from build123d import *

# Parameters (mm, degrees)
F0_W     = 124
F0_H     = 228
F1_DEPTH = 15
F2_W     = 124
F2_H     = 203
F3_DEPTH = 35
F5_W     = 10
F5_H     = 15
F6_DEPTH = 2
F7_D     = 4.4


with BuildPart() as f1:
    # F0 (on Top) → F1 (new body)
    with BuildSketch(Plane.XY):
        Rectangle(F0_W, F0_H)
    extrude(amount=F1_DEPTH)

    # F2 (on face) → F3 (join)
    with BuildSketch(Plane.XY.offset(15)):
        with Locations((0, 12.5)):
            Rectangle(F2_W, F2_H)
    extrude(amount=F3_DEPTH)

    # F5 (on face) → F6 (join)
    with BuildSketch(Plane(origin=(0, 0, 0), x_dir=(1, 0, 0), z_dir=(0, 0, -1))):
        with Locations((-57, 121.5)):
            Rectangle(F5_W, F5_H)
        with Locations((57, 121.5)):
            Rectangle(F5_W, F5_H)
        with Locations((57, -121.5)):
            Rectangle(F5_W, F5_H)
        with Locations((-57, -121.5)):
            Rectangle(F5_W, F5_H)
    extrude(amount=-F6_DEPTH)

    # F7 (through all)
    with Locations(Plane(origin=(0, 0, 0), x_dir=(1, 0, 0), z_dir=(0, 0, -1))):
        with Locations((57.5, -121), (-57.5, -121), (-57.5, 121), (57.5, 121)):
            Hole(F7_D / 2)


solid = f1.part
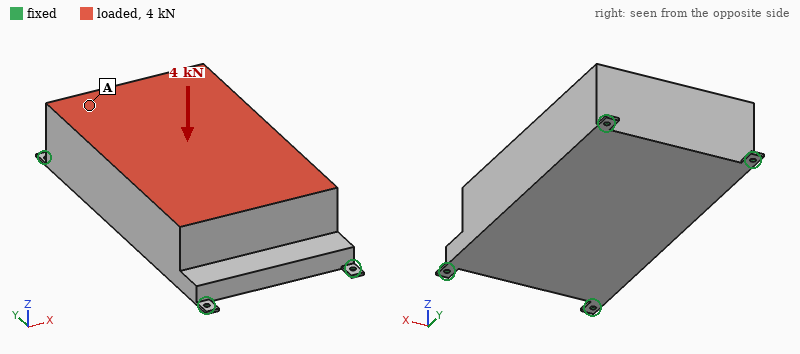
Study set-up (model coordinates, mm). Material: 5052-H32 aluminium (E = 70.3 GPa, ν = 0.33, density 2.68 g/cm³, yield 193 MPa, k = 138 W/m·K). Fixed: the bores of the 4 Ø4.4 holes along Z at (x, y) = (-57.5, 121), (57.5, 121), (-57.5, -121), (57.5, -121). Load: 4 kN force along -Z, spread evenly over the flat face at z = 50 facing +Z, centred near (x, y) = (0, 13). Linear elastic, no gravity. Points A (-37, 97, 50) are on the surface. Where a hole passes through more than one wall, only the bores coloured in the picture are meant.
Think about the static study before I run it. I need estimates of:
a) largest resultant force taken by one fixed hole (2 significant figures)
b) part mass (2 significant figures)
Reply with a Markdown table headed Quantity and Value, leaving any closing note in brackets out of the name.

| Quantity | Value |
|---|---|
| largest resultant force taken by one fixed hole | 1.4 kN |
| part mass | 3.5 kg |
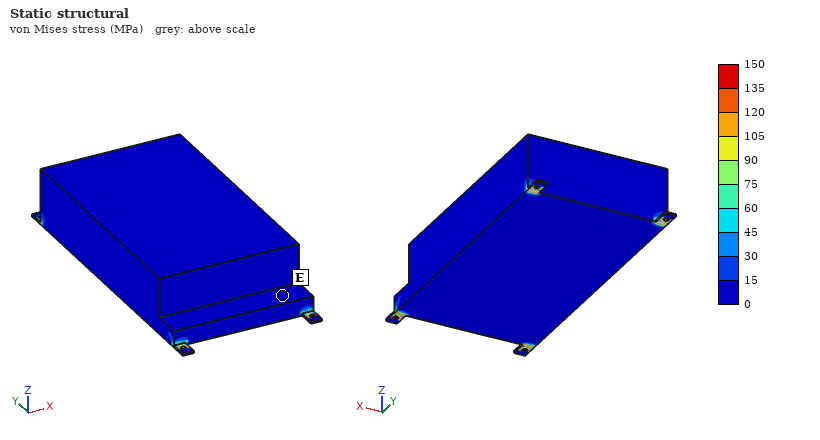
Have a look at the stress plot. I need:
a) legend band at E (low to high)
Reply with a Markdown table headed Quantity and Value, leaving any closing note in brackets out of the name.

| Quantity | Value |
|---|---|
| legend band at E | 0 to 15 MPa |
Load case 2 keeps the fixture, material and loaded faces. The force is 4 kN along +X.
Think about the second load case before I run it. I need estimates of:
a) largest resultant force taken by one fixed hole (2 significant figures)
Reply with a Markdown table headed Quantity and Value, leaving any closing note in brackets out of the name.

| Quantity | Value |
|---|---|
| largest resultant force taken by one fixed hole | 1.6 kN |
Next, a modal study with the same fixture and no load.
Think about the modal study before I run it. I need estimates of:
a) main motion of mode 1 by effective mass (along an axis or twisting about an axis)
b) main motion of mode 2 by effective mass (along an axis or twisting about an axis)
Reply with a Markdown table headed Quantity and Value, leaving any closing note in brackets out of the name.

| Quantity | Value |
|---|---|
| main motion of mode 1 by effective mass | along Z |
| main motion of mode 2 by effective mass | along X |
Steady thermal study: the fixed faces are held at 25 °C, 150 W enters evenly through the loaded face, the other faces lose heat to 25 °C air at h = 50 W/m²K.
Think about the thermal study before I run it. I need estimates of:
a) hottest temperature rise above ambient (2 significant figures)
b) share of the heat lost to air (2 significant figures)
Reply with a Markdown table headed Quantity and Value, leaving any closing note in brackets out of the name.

| Quantity | Value |
|---|---|
| hottest temperature rise above ambient | 37 K |
| share of the heat lost to air | 74 % |
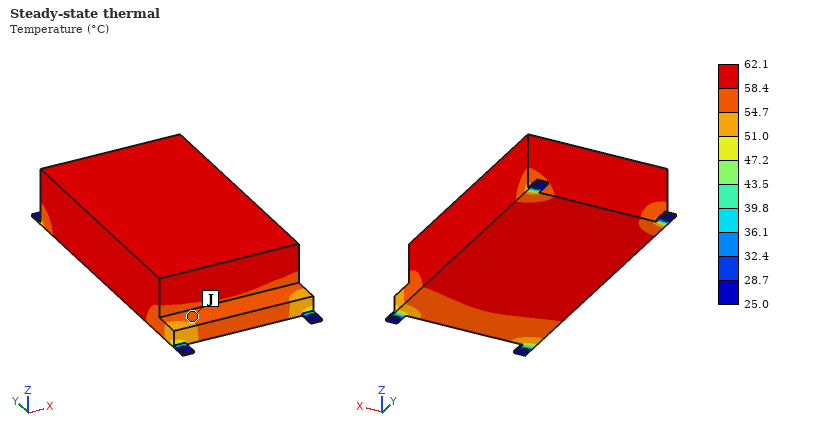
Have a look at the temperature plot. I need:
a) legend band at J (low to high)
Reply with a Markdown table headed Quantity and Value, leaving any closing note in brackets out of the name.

| Quantity | Value |
|---|---|
| legend band at J | 54.7 to 58.4 °C |
